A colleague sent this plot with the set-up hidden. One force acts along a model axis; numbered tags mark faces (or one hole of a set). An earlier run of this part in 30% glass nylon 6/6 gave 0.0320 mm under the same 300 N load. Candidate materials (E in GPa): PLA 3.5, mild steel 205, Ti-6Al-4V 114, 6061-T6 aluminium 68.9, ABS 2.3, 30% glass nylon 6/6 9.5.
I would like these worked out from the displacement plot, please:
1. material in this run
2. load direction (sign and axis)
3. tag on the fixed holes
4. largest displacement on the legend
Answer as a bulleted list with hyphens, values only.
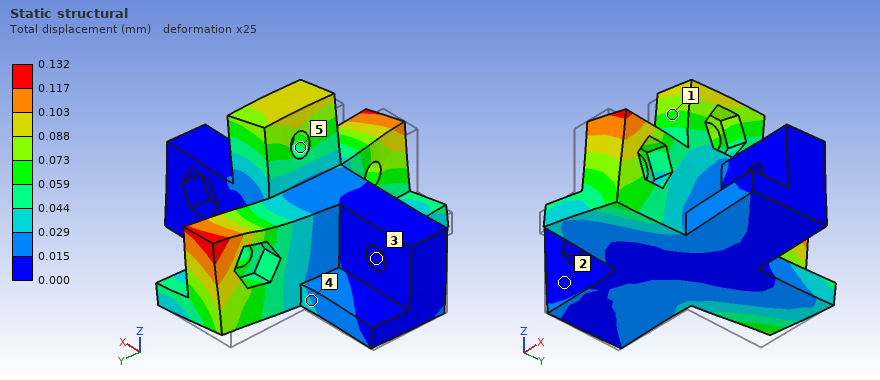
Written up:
- ABS
- +X
- 3
- 0.132 mm
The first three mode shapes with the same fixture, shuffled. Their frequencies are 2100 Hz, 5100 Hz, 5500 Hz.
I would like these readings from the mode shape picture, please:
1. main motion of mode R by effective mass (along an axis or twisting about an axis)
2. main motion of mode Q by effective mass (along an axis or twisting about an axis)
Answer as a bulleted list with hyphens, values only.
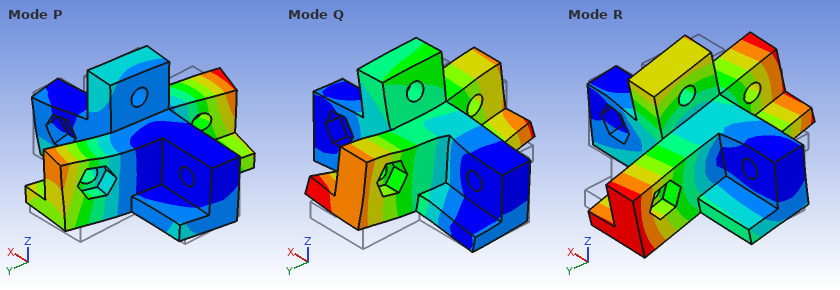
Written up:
- twisting about X
- along Z
